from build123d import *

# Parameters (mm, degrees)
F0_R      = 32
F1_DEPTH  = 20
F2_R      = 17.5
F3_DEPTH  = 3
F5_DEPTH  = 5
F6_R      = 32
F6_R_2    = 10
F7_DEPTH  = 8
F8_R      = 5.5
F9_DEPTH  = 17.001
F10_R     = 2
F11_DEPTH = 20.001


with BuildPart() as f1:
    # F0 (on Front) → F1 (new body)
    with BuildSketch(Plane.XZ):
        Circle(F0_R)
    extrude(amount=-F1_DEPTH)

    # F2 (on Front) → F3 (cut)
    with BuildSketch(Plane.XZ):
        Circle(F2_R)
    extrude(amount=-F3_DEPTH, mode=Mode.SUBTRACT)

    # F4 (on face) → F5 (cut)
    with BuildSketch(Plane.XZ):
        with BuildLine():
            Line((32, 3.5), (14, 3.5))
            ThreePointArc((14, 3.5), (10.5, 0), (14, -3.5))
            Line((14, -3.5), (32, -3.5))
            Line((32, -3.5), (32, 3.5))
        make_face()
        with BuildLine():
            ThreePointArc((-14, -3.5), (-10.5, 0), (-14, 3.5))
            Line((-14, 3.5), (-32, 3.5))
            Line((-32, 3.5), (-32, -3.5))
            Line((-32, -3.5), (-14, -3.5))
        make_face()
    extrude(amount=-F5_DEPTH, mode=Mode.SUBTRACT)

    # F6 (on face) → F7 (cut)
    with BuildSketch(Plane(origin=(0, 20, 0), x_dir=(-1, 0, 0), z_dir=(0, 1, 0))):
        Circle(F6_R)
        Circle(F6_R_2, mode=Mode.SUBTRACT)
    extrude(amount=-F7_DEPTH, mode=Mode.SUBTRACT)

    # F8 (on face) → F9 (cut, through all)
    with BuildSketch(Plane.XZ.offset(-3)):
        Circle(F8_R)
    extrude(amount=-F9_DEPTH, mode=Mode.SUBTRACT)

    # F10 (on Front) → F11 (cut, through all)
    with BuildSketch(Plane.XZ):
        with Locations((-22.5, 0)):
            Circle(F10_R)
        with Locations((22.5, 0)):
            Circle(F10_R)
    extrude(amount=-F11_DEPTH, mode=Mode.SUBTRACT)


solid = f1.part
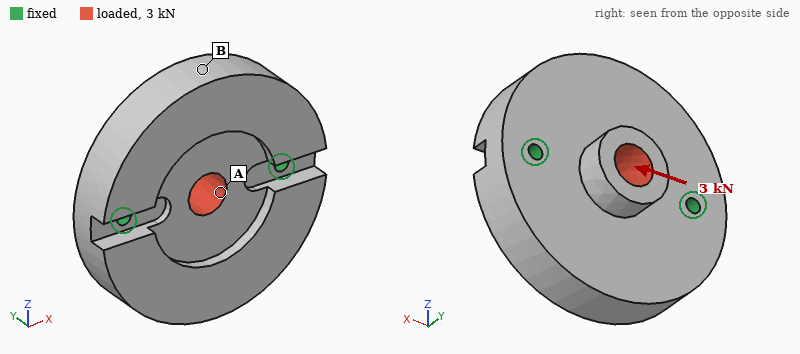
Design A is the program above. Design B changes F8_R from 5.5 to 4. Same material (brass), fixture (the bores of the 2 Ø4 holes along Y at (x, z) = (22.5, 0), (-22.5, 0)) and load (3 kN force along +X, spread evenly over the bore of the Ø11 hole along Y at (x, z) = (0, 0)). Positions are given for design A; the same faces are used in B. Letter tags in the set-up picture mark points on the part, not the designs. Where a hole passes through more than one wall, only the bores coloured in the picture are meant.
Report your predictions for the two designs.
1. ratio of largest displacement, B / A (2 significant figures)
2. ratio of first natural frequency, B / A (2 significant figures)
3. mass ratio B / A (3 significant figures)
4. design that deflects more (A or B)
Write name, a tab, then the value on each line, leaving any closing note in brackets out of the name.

ratio of largest displacement, B / A	0.91
ratio of first natural frequency, B / A	1.00
mass ratio B / A	1.02
design that deflects more	A
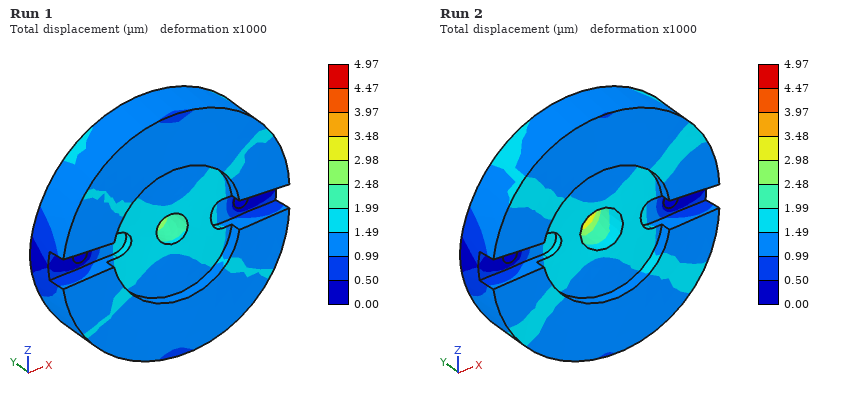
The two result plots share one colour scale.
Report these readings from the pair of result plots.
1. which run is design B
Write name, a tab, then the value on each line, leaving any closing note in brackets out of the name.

which run is design B	Run 1
